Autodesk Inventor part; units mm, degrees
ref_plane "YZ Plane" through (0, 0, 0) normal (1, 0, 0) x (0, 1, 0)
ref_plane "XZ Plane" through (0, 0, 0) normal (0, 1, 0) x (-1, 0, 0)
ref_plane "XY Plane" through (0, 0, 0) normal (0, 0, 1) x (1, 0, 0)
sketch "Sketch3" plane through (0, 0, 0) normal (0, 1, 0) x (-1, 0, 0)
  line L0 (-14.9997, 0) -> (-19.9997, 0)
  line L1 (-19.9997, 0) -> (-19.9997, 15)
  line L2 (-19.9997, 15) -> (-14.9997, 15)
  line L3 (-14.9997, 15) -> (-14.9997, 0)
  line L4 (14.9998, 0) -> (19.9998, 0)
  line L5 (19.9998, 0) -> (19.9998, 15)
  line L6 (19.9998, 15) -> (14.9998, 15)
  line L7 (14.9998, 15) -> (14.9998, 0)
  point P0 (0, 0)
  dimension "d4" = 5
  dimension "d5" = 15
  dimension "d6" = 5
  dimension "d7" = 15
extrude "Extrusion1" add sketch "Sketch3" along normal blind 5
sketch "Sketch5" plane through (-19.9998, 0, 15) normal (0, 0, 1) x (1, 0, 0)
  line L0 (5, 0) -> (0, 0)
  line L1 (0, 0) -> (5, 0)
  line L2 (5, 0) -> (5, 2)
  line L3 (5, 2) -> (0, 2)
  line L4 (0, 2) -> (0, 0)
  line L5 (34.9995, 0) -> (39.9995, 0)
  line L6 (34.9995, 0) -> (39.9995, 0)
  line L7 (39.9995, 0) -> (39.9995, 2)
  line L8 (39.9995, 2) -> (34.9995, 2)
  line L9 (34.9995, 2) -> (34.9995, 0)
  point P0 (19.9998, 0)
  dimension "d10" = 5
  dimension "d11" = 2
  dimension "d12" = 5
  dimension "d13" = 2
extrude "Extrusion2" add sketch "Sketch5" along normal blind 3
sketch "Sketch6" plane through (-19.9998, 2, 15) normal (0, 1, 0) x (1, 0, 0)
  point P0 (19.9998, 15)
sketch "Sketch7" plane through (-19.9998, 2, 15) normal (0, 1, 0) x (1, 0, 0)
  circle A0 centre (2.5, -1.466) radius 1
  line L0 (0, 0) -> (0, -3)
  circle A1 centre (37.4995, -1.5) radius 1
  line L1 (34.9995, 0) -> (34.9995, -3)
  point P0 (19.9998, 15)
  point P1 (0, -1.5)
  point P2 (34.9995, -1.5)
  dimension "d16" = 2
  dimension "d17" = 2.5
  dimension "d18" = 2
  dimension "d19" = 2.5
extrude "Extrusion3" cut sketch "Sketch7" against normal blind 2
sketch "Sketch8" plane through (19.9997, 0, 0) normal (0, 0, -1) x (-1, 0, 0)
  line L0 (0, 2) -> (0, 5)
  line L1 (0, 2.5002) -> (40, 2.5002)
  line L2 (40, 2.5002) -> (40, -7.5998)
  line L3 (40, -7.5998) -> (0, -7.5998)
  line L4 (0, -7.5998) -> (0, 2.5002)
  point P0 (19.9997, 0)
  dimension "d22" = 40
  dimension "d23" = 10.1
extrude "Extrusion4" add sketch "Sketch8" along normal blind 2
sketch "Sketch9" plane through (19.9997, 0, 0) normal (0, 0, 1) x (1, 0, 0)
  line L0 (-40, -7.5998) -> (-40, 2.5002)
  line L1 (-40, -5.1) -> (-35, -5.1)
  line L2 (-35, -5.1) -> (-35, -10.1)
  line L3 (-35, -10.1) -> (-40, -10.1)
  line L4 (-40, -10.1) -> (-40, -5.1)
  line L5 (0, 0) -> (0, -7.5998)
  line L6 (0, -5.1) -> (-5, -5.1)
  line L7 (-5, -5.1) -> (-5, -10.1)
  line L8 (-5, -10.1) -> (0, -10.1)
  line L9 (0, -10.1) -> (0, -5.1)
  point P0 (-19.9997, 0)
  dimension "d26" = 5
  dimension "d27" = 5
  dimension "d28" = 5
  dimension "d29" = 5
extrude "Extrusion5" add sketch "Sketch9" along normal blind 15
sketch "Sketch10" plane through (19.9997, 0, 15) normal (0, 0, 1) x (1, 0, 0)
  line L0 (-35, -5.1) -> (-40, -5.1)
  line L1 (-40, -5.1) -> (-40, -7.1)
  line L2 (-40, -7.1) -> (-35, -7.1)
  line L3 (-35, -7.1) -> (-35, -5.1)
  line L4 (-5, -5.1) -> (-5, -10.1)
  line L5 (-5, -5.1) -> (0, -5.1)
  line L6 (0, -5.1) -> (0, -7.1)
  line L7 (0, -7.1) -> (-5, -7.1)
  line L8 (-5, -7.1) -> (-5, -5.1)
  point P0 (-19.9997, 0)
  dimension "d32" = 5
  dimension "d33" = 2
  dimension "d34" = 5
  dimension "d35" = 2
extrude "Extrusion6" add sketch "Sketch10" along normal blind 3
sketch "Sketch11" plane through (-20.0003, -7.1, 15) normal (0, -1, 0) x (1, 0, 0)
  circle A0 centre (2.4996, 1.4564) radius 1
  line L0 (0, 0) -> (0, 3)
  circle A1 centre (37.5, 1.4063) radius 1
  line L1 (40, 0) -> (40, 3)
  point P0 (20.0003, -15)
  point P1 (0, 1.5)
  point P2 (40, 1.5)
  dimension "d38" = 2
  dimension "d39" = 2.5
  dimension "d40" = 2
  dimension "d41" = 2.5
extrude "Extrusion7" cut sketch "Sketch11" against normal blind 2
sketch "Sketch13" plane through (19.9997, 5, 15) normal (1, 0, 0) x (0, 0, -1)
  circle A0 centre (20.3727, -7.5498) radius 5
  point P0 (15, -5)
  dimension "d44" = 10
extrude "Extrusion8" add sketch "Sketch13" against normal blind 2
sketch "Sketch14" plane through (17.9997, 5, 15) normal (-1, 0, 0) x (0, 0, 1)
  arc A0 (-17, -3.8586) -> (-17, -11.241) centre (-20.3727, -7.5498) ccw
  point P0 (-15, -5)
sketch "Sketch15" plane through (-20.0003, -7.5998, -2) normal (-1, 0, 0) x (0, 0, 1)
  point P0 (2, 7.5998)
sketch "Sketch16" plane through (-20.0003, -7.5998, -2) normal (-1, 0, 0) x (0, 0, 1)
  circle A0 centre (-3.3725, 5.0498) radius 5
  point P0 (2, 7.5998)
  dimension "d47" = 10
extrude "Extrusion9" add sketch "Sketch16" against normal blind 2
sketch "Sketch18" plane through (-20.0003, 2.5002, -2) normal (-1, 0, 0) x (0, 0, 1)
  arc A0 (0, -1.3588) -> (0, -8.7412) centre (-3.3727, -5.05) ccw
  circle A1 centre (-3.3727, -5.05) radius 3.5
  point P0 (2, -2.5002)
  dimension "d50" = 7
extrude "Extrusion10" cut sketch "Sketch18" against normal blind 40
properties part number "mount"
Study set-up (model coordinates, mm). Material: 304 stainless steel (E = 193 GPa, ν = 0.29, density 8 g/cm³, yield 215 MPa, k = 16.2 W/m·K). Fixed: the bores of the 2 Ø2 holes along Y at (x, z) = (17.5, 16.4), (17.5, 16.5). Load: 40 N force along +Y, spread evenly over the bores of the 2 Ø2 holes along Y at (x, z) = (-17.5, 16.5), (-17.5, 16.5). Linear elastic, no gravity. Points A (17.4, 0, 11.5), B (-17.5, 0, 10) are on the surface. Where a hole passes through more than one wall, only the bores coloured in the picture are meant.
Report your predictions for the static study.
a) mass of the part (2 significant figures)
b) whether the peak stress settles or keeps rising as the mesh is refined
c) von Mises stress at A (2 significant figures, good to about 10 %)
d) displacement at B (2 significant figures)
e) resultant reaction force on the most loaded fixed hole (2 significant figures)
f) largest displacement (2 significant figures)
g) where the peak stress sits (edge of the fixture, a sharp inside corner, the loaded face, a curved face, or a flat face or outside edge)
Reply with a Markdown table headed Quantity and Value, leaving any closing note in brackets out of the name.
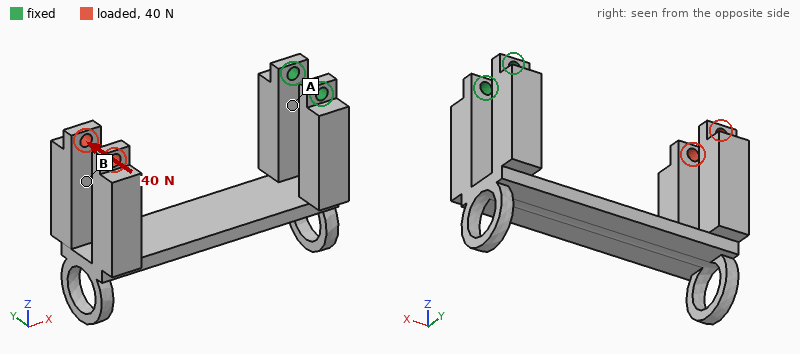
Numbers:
| Quantity | Value |
|---|---|
| mass of the part | 20 g |
| whether the peak stress settles or keeps rising as the mesh is refined | keeps rising |
| von Mises stress at A | 32 MPa |
| displacement at B | 0.25 mm |
| resultant reaction force on the most loaded fixed hole | 54 N |
| largest displacement | 0.37 mm |
| where the peak stress sits | edge of the fixture |
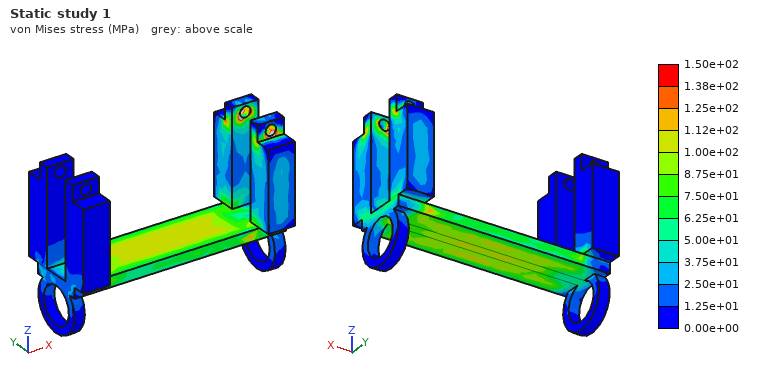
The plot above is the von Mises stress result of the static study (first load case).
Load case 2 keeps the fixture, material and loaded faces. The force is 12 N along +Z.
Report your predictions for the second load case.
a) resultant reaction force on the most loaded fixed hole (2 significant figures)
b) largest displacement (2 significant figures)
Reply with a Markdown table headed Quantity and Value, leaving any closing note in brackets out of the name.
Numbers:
| Quantity | Value |
|---|---|
| resultant reaction force on the most loaded fixed hole | 6.3 N |
| largest displacement | 0.19 mm |
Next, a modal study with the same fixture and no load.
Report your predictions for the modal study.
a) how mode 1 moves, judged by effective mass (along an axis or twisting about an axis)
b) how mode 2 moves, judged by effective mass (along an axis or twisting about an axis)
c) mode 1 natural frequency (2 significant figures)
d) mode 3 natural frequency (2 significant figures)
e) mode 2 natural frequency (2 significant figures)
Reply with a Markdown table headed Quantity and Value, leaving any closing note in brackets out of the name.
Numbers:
| Quantity | Value |
|---|---|
| how mode 1 moves, judged by effective mass | along Z |
| how mode 2 moves, judged by effective mass | along Y |
| mode 1 natural frequency | 470 Hz |
| mode 3 natural frequency | 1900 Hz |
| mode 2 natural frequency | 880 Hz |
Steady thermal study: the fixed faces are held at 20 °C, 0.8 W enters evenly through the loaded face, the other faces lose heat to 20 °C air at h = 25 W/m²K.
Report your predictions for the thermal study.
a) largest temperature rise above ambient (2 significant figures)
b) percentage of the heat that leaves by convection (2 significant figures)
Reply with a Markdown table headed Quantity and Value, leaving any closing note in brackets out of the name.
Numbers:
| Quantity | Value |
|---|---|
| largest temperature rise above ambient | 36 K |
| percentage of the heat that leaves by convection | 92 % |
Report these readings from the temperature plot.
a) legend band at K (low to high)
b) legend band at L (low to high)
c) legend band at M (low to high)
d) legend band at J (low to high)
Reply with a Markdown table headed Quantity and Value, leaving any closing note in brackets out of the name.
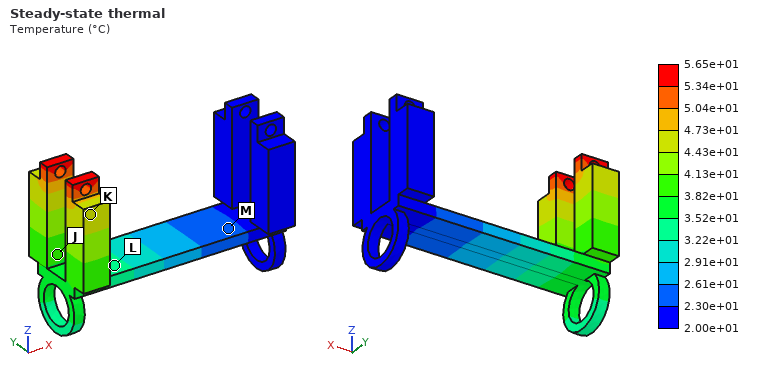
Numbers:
| Quantity | Value |
|---|---|
| legend band at K | 4.43e+01 to 4.73e+01 °C |
| legend band at L | 3.22e+01 to 3.52e+01 °C |
| legend band at M | 2.30e+01 to 2.61e+01 °C |
| legend band at J | 3.82e+01 to 4.13e+01 °C |
